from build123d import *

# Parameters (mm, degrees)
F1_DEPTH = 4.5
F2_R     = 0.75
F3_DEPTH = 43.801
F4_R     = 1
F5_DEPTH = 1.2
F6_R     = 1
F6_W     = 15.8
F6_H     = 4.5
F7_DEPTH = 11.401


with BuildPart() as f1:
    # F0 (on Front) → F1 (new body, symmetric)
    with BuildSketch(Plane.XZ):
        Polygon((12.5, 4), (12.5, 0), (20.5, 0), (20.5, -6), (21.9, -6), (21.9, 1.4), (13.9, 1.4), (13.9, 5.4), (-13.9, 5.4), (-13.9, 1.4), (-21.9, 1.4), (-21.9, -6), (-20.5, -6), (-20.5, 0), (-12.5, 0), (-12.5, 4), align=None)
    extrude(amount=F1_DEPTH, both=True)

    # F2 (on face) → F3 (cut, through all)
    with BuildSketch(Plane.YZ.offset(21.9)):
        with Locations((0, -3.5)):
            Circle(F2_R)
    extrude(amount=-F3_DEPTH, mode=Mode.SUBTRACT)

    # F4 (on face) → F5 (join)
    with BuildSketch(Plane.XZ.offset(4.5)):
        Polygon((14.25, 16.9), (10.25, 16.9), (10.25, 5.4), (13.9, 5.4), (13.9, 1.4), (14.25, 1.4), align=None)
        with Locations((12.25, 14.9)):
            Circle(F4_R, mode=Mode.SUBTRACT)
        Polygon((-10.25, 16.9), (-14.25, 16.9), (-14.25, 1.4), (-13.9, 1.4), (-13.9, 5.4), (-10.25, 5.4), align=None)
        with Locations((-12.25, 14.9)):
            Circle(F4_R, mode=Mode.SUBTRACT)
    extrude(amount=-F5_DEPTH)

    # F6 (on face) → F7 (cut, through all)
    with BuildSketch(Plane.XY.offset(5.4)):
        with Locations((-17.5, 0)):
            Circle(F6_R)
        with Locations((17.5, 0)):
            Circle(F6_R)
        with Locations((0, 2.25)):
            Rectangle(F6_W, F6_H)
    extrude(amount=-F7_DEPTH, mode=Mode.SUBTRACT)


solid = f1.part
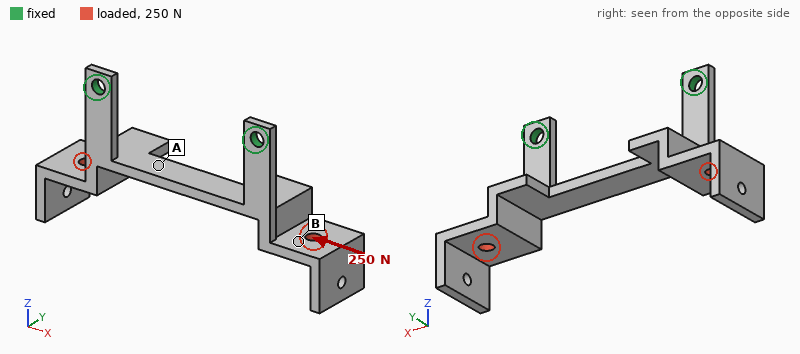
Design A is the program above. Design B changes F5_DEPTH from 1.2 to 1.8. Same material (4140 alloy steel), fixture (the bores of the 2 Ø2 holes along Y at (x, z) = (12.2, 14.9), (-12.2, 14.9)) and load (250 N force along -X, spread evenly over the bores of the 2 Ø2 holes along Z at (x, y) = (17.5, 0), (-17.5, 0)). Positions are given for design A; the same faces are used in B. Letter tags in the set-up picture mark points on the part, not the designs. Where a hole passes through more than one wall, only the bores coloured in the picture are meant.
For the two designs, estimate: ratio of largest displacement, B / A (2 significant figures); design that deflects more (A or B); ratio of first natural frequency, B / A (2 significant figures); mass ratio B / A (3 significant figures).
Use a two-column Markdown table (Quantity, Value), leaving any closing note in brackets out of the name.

| Quantity | Value |
|---|---|
| ratio of largest displacement, B / A | 0.71 |
| design that deflects more | A |
| ratio of first natural frequency, B / A | 1.8 |
| mass ratio B / A | 1.07 |
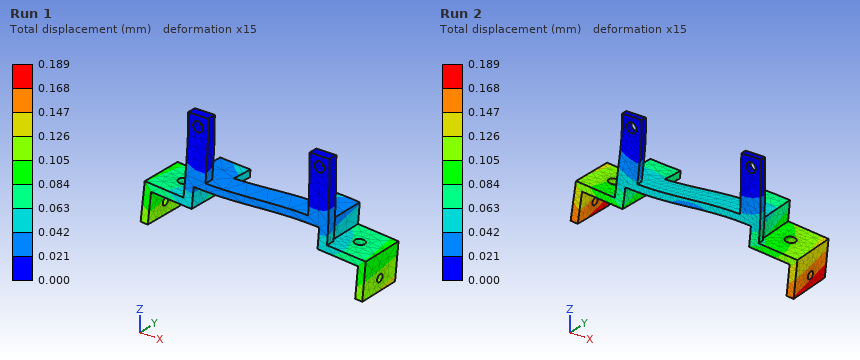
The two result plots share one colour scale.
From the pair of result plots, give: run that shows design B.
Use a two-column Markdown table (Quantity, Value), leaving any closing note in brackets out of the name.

| Quantity | Value |
|---|---|
| run that shows design B | Run 1 |
